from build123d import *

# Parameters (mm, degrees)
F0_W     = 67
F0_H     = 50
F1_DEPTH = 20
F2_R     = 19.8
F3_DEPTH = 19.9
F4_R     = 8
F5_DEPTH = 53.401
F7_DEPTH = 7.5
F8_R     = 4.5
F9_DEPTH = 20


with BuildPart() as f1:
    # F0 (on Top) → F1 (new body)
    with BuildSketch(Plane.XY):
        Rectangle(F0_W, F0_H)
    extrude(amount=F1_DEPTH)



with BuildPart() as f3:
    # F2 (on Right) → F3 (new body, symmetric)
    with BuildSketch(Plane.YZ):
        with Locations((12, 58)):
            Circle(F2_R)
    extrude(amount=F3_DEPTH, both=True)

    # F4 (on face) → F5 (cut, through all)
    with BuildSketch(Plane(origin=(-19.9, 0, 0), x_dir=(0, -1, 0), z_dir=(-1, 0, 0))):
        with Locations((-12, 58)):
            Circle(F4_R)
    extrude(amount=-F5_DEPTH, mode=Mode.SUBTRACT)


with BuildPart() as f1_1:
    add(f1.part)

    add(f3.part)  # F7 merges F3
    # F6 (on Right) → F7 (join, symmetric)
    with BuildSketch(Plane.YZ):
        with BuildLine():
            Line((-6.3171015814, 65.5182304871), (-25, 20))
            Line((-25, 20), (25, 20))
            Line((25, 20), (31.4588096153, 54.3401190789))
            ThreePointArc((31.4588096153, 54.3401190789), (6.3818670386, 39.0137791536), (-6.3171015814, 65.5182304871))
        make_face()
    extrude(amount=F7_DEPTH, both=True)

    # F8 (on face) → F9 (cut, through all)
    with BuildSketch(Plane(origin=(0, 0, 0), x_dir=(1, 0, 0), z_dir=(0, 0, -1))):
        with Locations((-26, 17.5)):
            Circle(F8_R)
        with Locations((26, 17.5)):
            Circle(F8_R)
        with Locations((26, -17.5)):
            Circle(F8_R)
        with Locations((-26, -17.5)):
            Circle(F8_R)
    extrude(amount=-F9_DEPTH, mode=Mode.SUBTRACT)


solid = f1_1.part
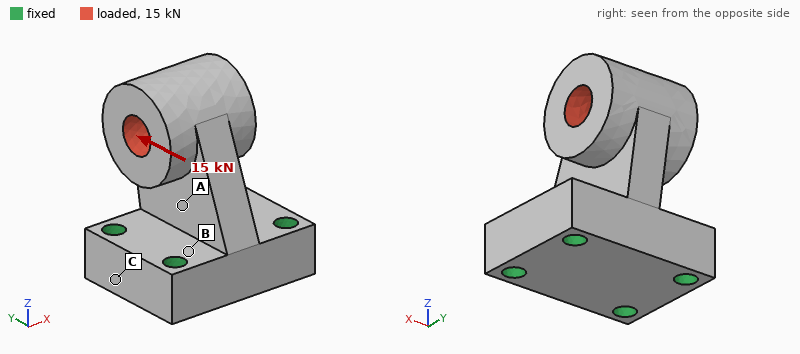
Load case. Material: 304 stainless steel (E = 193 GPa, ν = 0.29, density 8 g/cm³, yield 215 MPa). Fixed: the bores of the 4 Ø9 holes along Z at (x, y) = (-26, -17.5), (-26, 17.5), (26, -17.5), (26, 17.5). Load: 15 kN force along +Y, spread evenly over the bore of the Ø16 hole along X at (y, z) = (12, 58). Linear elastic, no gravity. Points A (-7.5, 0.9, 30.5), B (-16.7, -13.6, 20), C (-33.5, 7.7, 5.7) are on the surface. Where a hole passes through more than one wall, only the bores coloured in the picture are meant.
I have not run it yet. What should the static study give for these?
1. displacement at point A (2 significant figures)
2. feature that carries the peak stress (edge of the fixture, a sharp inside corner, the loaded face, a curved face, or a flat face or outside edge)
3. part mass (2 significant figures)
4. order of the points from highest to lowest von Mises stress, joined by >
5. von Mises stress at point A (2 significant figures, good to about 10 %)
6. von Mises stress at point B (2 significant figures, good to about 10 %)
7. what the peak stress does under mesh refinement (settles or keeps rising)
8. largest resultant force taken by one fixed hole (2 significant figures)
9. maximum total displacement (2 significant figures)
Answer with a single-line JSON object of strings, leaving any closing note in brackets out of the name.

{"displacement at point A": "18 µm", "feature that carries the peak stress": "edge of the fixture", "part mass": "960 g", "order of the points from highest to lowest von Mises stress, joined by >": "B > A > C", "von Mises stress at point A": "49 MPa", "von Mises stress at point B": "64 MPa", "what the peak stress does under mesh refinement": "keeps rising", "largest resultant force taken by one fixed hole": "10 kN", "maximum total displacement": "76 µm"}
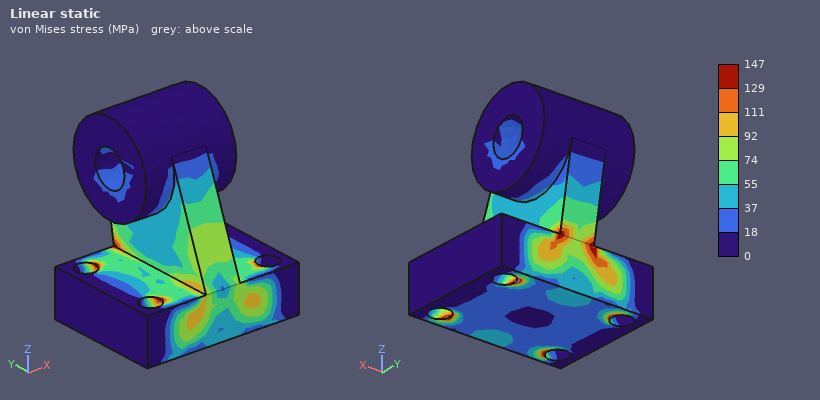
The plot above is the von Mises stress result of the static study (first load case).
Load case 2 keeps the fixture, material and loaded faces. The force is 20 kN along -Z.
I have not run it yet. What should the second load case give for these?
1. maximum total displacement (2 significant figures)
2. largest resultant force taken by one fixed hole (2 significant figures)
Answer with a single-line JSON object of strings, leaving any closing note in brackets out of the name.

{"maximum total displacement": "28 µm", "largest resultant force taken by one fixed hole": "8.1 kN"}
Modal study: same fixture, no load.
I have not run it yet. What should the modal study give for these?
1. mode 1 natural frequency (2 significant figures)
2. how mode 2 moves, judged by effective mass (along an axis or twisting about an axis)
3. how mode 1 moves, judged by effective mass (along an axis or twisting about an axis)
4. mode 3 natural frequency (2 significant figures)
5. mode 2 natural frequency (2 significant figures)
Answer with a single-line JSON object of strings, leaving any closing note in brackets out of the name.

{"mode 1 natural frequency": "2300 Hz", "how mode 2 moves, judged by effective mass": "along Y", "how mode 1 moves, judged by effective mass": "along X", "mode 3 natural frequency": "6500 Hz", "mode 2 natural frequency": "4200 Hz"}
